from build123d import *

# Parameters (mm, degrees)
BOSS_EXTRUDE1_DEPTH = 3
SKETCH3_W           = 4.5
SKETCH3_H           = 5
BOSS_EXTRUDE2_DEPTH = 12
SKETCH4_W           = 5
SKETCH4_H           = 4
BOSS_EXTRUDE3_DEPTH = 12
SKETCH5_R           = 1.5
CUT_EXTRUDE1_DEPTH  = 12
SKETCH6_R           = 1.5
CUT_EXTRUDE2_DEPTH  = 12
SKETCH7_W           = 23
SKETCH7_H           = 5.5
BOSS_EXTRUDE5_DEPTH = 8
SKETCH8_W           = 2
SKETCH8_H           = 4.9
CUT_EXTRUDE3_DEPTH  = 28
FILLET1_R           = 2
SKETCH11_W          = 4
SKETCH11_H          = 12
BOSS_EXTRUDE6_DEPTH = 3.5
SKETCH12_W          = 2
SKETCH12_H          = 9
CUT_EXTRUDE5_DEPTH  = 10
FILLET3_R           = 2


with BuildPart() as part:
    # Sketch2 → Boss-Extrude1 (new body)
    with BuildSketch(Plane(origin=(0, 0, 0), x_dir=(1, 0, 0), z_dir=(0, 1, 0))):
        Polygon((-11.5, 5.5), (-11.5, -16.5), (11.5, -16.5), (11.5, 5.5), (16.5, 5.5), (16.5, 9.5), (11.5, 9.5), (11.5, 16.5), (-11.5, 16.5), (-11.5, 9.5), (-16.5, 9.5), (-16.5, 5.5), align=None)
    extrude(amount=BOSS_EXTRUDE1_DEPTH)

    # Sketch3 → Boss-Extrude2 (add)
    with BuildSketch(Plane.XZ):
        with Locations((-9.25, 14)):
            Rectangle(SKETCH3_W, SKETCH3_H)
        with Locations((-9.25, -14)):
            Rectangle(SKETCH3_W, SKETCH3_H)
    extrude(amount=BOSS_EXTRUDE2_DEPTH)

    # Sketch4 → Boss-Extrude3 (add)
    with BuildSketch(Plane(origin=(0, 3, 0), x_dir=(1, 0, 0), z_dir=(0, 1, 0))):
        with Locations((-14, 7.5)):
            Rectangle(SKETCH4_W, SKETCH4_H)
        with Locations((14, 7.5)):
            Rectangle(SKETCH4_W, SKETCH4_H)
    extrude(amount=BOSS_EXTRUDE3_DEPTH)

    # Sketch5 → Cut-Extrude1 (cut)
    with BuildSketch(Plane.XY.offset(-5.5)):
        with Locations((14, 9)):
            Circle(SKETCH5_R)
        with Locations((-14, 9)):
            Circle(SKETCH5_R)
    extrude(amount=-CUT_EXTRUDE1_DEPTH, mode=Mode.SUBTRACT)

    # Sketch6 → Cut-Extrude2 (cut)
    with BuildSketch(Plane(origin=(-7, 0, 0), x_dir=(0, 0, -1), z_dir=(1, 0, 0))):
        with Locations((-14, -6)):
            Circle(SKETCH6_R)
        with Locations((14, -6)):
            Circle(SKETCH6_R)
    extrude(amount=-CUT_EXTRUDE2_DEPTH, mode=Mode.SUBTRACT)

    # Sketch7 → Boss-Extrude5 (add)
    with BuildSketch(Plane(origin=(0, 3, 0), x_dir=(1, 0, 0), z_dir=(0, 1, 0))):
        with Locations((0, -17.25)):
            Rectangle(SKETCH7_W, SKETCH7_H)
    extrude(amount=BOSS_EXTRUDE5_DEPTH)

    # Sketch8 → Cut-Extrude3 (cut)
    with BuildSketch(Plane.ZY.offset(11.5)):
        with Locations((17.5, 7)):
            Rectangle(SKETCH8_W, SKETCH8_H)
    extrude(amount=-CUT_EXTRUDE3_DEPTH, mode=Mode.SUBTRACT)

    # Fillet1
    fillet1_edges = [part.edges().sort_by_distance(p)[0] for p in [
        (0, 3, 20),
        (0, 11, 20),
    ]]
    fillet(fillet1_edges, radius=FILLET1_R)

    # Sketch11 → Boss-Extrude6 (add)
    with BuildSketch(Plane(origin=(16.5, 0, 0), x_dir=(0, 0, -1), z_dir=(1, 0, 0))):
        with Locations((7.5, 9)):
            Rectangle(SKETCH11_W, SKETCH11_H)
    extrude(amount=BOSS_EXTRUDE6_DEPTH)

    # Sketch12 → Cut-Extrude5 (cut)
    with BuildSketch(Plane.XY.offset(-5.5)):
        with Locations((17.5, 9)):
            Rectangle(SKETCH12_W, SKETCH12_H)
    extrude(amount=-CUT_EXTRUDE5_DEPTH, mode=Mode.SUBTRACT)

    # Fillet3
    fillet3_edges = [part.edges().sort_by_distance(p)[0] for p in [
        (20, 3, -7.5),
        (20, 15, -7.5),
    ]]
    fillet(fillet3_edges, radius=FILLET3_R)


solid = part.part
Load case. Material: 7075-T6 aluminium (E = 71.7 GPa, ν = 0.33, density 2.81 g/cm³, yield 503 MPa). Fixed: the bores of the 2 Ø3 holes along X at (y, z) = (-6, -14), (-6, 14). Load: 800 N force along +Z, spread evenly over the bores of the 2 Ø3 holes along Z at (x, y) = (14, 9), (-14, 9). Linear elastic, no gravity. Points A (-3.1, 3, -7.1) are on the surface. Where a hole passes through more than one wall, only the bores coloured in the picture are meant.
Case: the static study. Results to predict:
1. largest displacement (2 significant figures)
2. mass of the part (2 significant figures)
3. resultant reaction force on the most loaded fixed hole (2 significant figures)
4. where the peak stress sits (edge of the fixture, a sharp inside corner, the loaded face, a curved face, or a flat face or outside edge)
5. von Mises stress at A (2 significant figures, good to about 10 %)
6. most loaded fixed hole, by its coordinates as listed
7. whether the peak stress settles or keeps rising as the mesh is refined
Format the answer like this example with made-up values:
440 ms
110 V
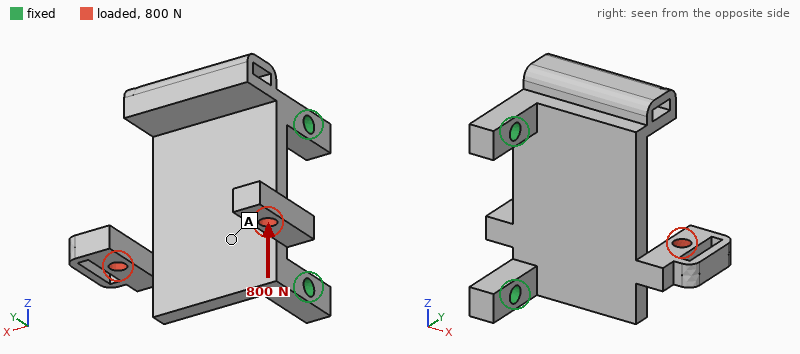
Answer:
0.35 mm
12 g
650 N
a sharp inside corner
38 MPa
(-6, 14)
keeps rising
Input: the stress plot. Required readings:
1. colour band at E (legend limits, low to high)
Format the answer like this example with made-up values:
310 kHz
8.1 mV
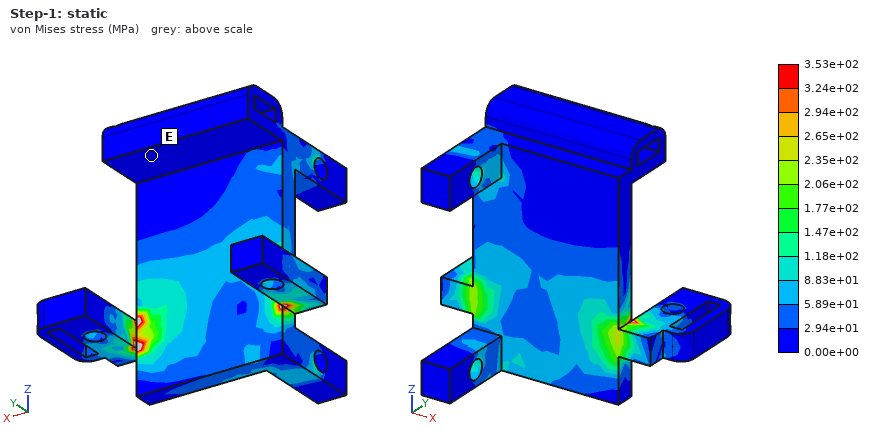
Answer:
0.00e+00 to 2.94e+01 MPa
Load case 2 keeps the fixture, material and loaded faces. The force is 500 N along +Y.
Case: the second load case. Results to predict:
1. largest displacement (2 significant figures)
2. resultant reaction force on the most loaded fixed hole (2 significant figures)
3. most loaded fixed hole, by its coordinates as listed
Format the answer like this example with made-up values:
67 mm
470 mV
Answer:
0.58 mm
440 N
(-6, -14)
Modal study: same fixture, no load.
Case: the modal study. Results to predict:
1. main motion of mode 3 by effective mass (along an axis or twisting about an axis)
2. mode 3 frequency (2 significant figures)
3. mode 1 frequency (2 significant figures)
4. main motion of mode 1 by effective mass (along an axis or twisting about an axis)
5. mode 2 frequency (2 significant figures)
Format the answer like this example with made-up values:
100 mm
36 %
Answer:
along Z
6800 Hz
2400 Hz
along Y
4900 Hz
